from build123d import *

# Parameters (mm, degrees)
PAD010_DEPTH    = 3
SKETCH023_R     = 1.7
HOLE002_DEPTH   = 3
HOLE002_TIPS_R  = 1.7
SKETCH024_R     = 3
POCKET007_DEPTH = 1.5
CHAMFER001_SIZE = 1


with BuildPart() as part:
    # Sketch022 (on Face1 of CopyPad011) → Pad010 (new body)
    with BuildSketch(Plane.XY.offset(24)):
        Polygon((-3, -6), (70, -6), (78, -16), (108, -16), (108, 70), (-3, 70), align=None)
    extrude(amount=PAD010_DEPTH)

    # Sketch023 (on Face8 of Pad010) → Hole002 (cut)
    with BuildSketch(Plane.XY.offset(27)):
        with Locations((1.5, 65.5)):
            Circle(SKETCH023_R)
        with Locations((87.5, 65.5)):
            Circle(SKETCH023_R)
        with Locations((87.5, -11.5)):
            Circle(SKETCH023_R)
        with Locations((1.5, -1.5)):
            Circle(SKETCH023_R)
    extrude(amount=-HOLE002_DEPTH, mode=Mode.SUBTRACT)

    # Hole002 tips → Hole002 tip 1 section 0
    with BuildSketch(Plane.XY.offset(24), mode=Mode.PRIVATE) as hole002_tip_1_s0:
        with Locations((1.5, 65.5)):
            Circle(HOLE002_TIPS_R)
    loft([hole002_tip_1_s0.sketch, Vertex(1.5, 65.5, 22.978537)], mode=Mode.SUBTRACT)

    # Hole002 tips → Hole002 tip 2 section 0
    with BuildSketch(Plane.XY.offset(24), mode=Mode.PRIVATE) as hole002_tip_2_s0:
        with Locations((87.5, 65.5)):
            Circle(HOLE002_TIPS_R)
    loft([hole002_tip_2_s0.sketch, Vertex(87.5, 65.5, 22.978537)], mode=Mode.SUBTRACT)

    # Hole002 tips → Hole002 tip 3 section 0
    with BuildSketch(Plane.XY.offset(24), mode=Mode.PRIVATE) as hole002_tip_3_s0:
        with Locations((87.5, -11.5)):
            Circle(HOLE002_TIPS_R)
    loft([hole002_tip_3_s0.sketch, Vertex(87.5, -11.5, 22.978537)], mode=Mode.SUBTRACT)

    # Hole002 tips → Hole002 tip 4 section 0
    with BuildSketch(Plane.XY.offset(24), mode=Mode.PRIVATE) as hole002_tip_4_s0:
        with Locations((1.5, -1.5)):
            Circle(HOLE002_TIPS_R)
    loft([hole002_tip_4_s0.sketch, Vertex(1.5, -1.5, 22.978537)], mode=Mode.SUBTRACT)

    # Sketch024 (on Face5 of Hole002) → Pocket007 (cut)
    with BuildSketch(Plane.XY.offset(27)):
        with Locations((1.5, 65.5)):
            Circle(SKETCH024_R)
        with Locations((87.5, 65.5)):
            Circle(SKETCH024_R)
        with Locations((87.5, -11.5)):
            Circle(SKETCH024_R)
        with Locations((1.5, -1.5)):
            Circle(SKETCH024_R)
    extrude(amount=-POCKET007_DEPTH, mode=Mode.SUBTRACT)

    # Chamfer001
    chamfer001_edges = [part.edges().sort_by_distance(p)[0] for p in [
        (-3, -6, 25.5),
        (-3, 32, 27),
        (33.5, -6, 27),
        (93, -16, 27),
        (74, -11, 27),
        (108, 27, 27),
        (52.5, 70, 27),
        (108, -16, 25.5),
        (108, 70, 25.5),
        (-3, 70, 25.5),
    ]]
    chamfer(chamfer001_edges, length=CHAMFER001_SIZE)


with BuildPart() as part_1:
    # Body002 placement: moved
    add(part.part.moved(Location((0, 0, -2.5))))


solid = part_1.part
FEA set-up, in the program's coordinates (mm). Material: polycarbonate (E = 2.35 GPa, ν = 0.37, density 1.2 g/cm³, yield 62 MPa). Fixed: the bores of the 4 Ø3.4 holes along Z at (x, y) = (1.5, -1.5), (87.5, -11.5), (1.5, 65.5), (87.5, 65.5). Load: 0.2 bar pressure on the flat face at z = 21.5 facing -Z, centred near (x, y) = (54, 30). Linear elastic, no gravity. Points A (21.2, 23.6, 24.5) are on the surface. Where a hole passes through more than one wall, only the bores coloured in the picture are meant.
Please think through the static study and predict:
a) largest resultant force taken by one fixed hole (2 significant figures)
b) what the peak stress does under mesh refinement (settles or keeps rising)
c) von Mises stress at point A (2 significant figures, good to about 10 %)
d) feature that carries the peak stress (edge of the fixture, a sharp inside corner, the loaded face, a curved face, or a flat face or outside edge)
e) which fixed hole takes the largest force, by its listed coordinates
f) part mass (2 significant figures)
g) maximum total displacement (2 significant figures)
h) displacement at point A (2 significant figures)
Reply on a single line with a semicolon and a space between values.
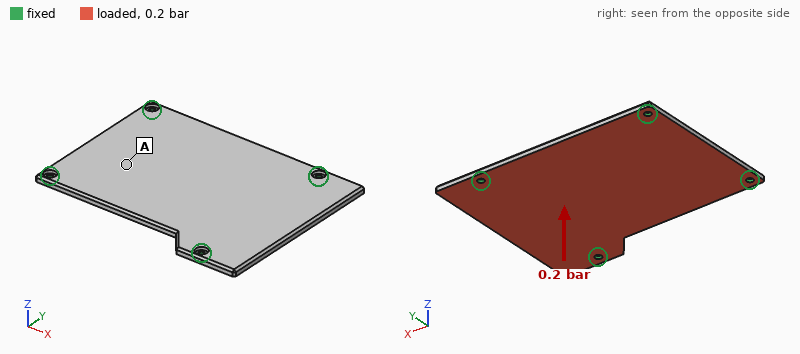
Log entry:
110 N; keeps rising; 4.4 MPa; edge of the fixture; (87.5, 65.5); 31 g; 1.4 mm; 0.98 mm
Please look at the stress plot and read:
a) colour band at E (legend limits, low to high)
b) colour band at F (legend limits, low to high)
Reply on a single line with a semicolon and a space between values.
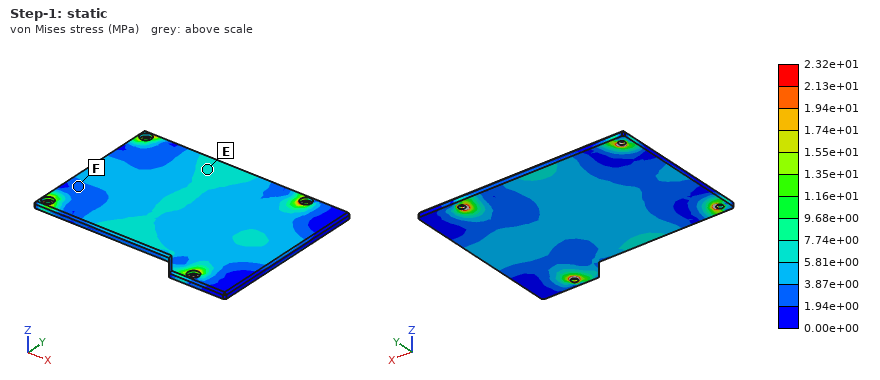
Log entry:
5.81e+00 to 7.74e+00 MPa; 1.94e+00 to 3.87e+00 MPa
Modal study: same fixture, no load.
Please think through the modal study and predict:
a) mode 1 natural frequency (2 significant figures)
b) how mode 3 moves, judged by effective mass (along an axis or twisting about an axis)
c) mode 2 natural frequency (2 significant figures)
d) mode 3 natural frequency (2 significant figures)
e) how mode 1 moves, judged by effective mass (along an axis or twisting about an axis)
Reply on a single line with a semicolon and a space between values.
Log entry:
370 Hz; twisting about X; 530 Hz; 640 Hz; along Z
